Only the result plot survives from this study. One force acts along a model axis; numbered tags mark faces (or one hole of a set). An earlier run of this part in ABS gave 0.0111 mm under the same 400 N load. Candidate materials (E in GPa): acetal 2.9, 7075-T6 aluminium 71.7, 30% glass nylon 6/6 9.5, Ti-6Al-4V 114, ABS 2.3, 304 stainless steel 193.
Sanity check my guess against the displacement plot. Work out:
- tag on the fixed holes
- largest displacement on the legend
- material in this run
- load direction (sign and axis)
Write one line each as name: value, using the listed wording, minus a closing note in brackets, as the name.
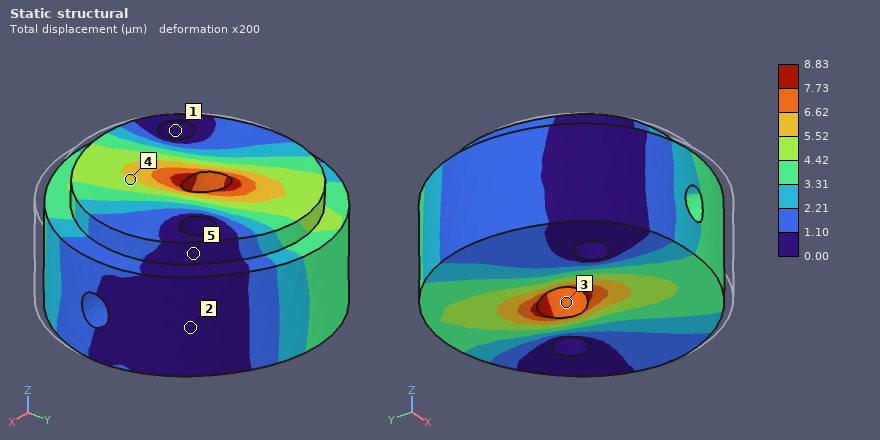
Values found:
tag on the fixed holes: 1
largest displacement on the legend: 8.83 µm
material in this run: acetal
load direction: +Y
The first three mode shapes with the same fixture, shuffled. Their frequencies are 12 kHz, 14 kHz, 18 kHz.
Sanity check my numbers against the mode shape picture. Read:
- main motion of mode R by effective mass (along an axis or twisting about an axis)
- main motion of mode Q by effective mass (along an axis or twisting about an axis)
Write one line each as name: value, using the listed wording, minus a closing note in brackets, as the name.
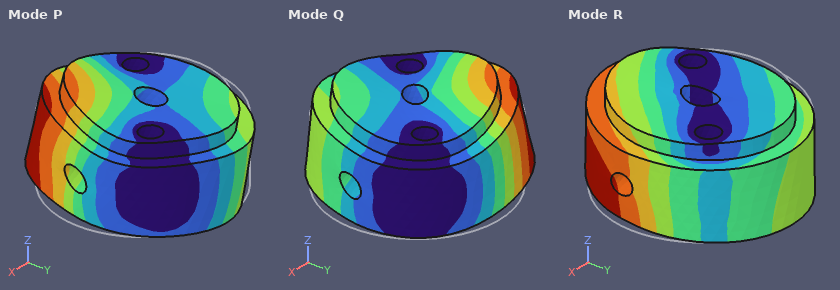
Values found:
main motion of mode R by effective mass: twisting about Z
main motion of mode Q by effective mass: along Z
